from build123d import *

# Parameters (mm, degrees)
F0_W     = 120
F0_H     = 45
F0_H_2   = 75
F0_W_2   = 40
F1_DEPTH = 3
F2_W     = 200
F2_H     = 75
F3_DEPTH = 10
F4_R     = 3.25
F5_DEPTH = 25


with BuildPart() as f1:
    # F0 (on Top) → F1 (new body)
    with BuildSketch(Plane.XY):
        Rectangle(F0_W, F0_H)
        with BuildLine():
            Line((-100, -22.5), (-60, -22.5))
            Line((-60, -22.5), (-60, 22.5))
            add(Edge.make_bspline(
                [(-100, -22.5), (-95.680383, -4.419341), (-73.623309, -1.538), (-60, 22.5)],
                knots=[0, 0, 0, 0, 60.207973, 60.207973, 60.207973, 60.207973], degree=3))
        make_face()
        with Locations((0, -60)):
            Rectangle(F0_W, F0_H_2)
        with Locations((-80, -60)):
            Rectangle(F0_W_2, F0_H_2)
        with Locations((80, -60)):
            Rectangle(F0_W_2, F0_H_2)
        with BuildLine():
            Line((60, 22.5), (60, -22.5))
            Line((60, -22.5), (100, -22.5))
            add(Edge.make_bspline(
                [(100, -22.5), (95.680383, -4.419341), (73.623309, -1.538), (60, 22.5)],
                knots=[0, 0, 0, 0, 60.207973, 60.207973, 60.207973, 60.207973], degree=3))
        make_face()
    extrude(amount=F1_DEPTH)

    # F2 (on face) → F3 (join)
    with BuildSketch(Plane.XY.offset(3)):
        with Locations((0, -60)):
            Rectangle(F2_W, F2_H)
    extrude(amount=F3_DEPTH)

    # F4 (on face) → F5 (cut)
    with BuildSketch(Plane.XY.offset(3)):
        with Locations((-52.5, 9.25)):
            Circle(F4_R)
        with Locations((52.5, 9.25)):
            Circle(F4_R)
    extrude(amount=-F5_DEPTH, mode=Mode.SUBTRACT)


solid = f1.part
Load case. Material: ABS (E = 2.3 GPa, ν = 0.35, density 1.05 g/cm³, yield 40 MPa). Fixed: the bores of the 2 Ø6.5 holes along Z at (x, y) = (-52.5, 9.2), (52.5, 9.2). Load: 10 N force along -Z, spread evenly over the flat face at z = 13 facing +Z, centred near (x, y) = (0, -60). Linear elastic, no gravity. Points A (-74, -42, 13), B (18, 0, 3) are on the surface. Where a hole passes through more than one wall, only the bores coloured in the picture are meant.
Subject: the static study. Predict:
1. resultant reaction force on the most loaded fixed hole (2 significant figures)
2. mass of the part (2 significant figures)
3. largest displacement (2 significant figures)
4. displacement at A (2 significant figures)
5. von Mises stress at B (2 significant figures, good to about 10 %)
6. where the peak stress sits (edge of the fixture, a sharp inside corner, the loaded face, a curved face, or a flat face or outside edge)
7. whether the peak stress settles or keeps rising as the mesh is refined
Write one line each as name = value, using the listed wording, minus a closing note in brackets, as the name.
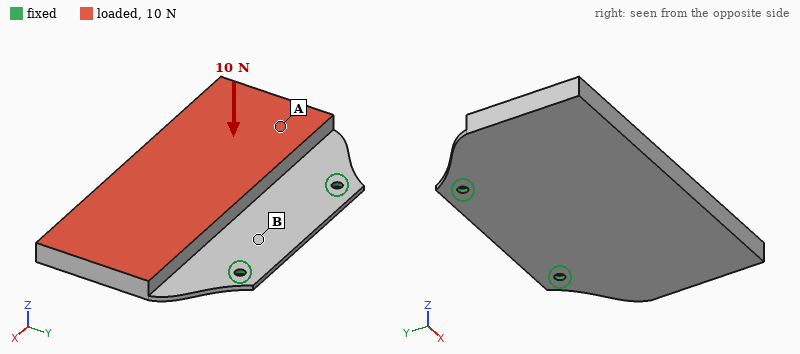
resultant reaction force on the most loaded fixed hole = 5.0 N
mass of the part = 230 g
largest displacement = 2.4 mm
displacement at A = 1.0 mm
von Mises stress at B = 1.2 MPa
where the peak stress sits = edge of the fixture
whether the peak stress settles or keeps rising as the mesh is refined = keeps rising
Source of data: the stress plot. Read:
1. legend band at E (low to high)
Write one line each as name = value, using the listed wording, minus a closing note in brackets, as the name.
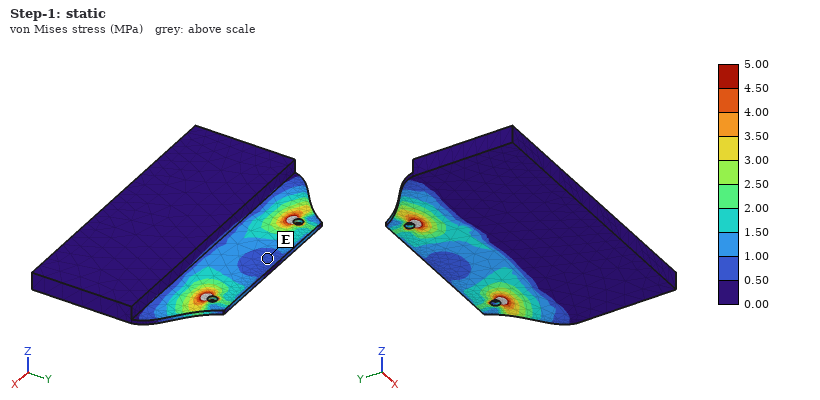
legend band at E = 0.50 to 1.00 MPa
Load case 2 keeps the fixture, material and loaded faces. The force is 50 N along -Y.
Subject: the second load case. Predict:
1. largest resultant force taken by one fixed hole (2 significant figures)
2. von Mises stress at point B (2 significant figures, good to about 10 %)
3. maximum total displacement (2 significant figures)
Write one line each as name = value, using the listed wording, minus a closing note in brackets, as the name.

largest resultant force taken by one fixed hole = 25 N
von Mises stress at point B = 1.4 MPa
maximum total displacement = 2.5 mm
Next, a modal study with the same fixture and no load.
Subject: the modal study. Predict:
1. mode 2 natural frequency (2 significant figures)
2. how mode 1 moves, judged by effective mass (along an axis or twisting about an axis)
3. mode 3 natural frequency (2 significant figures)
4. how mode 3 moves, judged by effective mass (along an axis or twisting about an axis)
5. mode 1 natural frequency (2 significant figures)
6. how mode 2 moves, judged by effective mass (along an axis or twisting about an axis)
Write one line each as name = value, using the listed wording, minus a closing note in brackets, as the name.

mode 2 natural frequency = 120 Hz
how mode 1 moves, judged by effective mass = along Z
mode 3 natural frequency = 350 Hz
how mode 3 moves, judged by effective mass = along Z
mode 1 natural frequency = 27 Hz
how mode 2 moves, judged by effective mass = twisting about Y
